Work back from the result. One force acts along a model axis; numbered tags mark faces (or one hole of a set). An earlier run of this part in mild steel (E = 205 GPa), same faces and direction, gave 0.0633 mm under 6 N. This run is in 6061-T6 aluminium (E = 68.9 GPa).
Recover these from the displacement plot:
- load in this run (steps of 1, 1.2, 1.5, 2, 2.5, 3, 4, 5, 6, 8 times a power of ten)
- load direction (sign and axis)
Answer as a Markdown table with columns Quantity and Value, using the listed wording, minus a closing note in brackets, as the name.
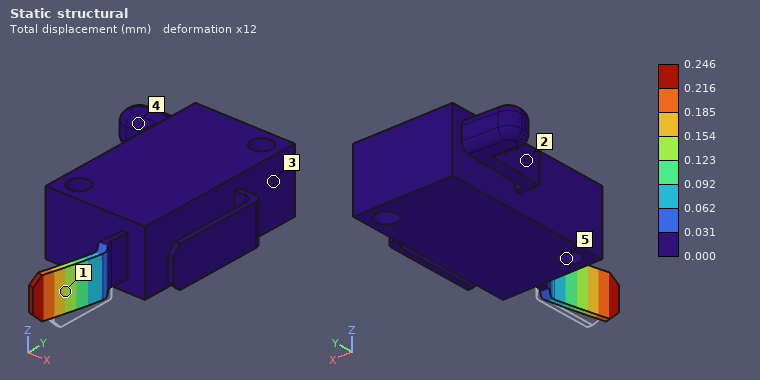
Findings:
| Quantity | Value |
|---|---|
| load in this run | 8 N |
| load direction | -X |
